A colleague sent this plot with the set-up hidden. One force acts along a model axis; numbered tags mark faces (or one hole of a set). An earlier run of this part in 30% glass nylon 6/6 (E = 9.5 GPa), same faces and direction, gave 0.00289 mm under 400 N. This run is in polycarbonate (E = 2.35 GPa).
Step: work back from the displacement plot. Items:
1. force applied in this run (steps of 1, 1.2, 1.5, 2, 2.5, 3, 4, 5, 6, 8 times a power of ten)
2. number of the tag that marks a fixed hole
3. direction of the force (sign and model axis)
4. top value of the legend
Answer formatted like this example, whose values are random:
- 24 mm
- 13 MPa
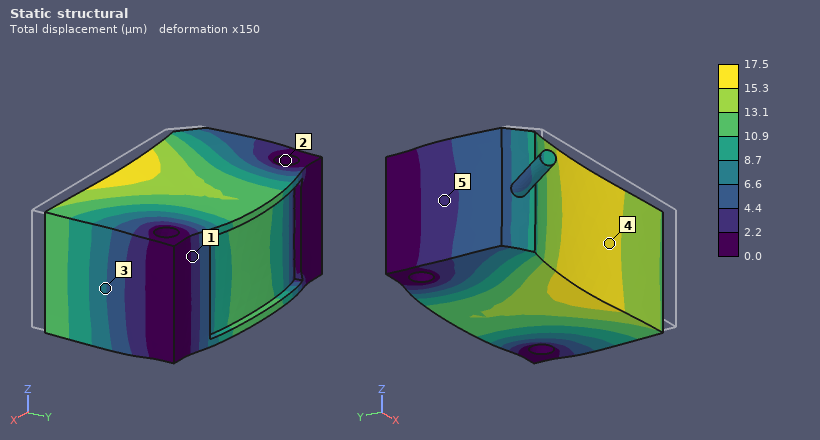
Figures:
- 600 N
- 2
- +Y
- 17.5 µm
